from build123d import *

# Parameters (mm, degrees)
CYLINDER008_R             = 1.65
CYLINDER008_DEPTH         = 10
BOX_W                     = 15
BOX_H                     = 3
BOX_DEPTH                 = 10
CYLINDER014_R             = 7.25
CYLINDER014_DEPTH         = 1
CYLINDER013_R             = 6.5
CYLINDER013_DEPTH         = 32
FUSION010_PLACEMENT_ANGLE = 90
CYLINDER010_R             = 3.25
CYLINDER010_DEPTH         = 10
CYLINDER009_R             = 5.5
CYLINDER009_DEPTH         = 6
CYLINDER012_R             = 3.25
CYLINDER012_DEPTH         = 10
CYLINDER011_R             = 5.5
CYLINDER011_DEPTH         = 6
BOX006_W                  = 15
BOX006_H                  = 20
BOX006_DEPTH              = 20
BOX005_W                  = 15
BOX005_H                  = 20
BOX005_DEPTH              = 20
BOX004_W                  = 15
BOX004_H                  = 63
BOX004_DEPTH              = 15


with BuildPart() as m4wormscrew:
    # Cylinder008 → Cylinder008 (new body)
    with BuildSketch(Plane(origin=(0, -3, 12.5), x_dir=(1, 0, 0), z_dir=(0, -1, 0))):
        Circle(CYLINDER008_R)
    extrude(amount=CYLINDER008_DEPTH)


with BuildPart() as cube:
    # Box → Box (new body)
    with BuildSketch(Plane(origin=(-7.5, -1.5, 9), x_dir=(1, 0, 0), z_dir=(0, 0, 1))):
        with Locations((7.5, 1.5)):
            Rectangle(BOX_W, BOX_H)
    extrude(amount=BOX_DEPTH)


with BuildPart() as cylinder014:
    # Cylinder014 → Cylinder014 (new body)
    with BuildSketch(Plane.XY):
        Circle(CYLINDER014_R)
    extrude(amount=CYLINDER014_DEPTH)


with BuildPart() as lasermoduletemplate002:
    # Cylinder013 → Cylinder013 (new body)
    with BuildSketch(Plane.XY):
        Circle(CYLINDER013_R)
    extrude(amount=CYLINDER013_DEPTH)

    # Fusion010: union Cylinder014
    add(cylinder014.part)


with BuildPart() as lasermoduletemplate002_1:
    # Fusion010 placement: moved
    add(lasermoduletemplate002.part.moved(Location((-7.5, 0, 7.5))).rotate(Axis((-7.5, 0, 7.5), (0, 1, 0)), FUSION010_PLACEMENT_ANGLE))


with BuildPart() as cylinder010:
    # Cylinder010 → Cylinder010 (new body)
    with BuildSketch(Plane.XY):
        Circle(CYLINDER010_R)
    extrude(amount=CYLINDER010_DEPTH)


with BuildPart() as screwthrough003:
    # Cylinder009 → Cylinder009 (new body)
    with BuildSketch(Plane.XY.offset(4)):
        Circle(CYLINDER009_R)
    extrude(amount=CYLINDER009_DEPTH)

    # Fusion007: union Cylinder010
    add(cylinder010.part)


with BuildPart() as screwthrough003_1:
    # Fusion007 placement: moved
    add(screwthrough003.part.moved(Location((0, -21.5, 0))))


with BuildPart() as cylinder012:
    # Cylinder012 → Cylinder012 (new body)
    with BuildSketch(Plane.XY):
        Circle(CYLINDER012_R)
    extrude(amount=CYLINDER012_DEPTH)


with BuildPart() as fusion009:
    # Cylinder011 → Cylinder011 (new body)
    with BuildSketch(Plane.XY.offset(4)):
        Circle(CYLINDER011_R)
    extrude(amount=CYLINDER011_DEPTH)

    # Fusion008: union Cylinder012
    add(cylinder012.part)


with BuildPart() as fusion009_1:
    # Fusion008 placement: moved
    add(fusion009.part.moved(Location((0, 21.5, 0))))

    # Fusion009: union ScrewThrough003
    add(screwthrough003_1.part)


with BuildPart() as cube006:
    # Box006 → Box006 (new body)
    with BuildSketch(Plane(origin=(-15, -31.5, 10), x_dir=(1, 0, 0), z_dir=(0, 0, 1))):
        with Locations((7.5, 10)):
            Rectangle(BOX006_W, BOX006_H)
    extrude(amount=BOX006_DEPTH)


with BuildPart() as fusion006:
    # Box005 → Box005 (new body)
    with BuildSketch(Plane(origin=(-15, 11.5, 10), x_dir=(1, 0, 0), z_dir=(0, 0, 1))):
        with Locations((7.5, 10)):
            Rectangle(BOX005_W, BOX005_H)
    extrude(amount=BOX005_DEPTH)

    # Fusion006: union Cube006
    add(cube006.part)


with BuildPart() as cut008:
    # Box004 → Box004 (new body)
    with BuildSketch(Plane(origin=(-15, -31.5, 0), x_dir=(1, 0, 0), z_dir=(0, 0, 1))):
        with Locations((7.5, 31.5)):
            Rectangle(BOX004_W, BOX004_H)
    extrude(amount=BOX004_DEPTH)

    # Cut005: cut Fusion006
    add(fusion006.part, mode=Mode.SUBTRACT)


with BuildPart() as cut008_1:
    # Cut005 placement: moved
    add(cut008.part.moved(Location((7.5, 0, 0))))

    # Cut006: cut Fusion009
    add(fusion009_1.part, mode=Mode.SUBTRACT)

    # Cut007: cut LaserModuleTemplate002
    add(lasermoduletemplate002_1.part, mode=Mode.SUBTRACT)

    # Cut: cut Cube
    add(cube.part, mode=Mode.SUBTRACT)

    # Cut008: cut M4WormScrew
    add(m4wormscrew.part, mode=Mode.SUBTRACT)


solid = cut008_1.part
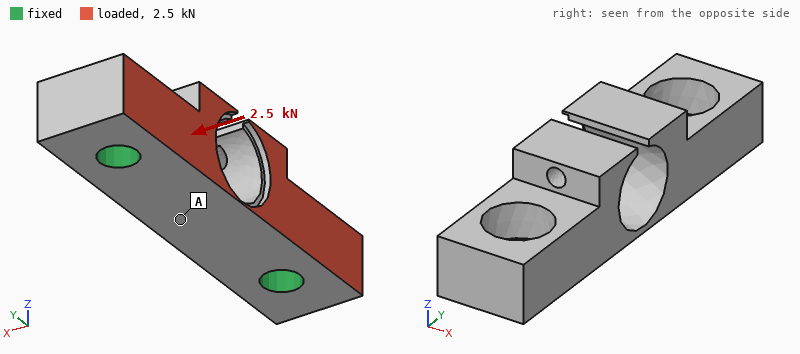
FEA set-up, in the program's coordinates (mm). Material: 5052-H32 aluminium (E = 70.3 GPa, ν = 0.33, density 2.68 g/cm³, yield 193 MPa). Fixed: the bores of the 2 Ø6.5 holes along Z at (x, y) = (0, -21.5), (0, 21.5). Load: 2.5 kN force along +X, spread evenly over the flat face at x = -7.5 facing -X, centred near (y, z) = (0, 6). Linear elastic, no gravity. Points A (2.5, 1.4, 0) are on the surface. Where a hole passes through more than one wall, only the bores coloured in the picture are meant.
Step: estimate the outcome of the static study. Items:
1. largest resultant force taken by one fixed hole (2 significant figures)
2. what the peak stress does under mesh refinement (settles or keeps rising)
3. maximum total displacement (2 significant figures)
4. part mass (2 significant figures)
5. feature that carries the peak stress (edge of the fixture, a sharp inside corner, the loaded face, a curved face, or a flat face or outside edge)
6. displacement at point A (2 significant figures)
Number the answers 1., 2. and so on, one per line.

1. 1.3 kN
2. keeps rising
3. 21 µm
4. 20 g
5. edge of the fixture
6. 7.0 µm
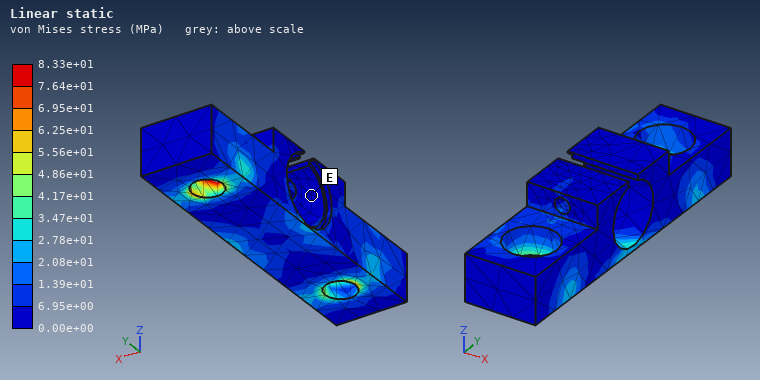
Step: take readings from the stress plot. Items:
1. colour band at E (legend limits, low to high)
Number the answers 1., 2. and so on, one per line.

1. 0.00e+00 to 6.95e+00 MPa
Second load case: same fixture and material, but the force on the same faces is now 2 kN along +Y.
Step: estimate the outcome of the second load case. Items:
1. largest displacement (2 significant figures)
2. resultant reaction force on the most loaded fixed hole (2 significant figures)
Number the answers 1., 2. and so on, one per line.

1. 16 µm
2. 1.0 kN
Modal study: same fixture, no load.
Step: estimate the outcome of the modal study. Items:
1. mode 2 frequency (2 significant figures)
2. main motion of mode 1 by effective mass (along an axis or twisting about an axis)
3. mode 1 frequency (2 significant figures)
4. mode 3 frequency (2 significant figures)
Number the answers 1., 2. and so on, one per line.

1. 15 kHz
2. along Z
3. 11 kHz
4. 15 kHz
